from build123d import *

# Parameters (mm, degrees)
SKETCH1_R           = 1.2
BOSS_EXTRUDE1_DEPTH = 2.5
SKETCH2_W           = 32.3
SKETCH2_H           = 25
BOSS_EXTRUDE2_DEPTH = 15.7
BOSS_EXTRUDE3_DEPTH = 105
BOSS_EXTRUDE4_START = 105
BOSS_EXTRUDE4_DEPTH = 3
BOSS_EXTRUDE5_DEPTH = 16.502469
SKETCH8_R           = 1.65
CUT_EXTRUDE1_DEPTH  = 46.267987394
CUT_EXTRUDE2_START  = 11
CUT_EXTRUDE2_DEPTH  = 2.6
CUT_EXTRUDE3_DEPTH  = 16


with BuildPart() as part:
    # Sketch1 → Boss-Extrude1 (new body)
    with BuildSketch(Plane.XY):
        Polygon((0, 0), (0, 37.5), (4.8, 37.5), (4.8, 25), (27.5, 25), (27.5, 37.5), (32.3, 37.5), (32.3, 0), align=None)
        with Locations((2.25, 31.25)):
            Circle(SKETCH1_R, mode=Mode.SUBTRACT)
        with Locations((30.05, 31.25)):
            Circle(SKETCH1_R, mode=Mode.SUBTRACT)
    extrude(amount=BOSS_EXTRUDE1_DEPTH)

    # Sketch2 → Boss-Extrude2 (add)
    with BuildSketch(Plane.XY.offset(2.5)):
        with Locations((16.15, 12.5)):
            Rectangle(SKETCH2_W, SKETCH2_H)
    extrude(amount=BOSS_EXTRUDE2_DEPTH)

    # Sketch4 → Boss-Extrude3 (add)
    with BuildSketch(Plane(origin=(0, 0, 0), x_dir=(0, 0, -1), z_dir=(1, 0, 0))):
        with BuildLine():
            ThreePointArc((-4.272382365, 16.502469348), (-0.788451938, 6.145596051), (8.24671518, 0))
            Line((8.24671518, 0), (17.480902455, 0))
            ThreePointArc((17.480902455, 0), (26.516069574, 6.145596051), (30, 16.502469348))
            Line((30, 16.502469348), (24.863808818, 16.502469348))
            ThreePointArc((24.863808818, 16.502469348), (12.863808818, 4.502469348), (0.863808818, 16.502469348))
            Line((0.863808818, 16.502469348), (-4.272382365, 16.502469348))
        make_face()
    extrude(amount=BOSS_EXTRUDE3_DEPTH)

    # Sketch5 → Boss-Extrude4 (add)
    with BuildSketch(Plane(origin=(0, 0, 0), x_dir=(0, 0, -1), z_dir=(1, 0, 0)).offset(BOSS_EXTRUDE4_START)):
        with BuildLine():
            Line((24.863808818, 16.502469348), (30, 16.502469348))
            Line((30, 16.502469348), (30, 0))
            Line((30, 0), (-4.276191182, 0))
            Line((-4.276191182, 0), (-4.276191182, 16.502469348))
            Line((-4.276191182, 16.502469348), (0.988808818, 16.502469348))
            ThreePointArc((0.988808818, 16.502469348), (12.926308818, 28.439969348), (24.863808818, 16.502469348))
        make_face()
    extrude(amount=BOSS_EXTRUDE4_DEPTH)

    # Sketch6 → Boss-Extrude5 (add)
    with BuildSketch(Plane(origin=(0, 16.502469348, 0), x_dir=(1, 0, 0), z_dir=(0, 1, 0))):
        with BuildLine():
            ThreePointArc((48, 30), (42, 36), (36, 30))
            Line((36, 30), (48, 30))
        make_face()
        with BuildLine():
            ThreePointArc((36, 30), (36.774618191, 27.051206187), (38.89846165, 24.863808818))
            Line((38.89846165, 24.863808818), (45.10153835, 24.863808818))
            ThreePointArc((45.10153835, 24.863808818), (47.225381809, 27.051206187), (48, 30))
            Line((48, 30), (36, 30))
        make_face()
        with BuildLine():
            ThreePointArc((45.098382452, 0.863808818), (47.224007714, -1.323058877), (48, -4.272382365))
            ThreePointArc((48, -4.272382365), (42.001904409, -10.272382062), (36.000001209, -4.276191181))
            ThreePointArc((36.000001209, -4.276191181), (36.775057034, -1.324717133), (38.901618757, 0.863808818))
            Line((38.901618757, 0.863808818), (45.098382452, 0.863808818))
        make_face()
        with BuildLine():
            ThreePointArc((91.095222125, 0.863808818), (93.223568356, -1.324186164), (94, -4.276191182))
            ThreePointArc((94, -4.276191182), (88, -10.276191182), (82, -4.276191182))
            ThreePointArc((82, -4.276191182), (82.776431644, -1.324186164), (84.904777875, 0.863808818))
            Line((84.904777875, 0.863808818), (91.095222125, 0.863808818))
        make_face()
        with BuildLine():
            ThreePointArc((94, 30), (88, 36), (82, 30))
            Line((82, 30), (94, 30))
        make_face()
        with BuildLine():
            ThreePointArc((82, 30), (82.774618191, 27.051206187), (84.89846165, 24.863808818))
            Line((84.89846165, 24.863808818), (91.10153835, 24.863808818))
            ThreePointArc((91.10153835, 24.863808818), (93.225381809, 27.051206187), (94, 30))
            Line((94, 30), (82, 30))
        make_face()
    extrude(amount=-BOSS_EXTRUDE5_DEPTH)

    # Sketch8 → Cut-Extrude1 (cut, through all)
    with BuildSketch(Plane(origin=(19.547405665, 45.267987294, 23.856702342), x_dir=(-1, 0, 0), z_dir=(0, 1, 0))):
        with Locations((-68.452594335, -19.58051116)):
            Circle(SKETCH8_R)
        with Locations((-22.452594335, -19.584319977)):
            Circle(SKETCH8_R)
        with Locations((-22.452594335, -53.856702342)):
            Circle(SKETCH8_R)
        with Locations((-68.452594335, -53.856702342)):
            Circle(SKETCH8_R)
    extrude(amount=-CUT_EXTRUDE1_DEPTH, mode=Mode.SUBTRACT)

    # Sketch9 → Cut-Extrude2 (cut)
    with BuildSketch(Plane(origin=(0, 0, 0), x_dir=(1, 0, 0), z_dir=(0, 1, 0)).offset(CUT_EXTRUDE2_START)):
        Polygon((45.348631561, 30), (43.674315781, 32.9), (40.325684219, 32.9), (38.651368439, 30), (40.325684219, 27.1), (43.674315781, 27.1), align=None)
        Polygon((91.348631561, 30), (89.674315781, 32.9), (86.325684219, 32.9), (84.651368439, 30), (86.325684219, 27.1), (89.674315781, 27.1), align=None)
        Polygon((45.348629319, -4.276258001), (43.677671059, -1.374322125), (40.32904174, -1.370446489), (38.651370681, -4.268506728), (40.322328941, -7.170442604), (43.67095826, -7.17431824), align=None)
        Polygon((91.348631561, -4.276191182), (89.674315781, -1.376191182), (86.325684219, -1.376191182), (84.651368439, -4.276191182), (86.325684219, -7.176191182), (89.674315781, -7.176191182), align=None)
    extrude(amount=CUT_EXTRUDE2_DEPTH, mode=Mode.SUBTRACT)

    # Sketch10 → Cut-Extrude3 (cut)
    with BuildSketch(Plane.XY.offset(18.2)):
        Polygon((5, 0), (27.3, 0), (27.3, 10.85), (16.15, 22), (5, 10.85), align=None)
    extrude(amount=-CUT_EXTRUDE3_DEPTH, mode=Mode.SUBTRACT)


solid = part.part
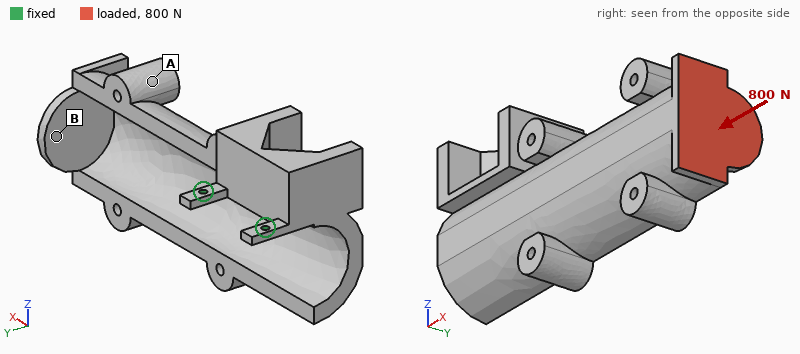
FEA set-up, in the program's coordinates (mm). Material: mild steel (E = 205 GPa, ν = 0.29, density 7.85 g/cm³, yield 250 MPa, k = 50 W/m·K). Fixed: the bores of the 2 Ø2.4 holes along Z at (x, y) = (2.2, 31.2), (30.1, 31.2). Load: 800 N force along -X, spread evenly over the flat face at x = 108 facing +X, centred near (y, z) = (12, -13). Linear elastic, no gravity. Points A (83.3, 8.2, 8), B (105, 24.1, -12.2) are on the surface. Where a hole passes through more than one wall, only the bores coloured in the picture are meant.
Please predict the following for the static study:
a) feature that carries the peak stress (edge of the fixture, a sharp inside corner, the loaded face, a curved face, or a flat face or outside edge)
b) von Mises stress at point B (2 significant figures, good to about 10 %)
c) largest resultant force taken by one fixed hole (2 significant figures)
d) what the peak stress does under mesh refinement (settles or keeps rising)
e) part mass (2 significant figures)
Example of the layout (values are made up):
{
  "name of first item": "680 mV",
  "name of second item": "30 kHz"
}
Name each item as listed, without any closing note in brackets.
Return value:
{
  "feature that carries the peak stress": "edge of the fixture",
  "von Mises stress at point B": "23 MPa",
  "largest resultant force taken by one fixed hole": "720 N",
  "what the peak stress does under mesh refinement": "keeps rising",
  "part mass": "310 g"
}
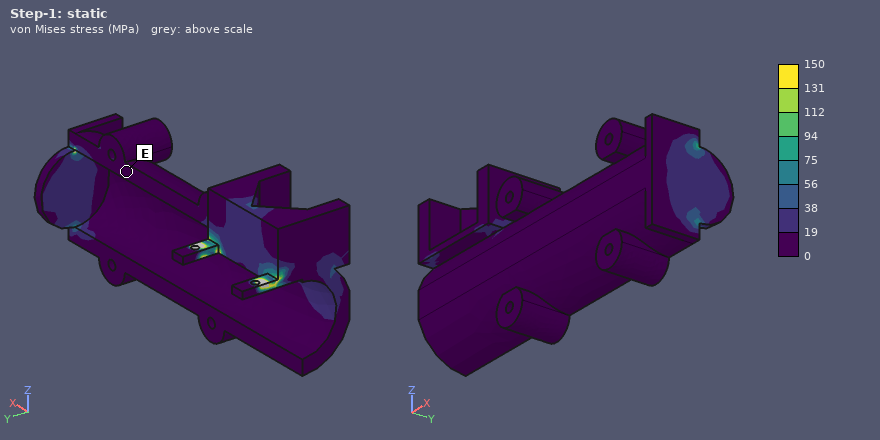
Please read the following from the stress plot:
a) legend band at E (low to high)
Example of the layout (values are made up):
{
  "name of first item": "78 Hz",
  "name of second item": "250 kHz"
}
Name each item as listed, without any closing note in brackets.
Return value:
{
  "legend band at E": "0 to 19 MPa"
}
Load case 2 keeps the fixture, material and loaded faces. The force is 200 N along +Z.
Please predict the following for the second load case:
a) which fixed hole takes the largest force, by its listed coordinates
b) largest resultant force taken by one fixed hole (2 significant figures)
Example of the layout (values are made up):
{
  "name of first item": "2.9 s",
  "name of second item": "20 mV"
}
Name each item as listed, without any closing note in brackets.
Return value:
{
  "which fixed hole takes the largest force, by its listed coordinates": "(30.1, 31.2)",
  "largest resultant force taken by one fixed hole": "750 N"
}
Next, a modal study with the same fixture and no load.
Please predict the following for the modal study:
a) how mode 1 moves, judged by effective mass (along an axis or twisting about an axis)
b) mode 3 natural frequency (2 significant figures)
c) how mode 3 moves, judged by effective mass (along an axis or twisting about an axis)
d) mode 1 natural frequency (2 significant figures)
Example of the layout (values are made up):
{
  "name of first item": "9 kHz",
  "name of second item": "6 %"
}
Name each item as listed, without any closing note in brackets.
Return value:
{
  "how mode 1 moves, judged by effective mass": "along Z",
  "mode 3 natural frequency": "940 Hz",
  "how mode 3 moves, judged by effective mass": "along Y",
  "mode 1 natural frequency": "210 Hz"
}
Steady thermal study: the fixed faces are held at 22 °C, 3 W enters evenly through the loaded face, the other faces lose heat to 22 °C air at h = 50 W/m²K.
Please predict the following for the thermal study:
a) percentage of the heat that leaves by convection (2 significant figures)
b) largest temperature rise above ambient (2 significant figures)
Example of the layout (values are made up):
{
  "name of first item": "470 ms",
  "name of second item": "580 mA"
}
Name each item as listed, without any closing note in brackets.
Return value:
{
  "percentage of the heat that leaves by convection": "96 %",
  "largest temperature rise above ambient": "12 K"
}
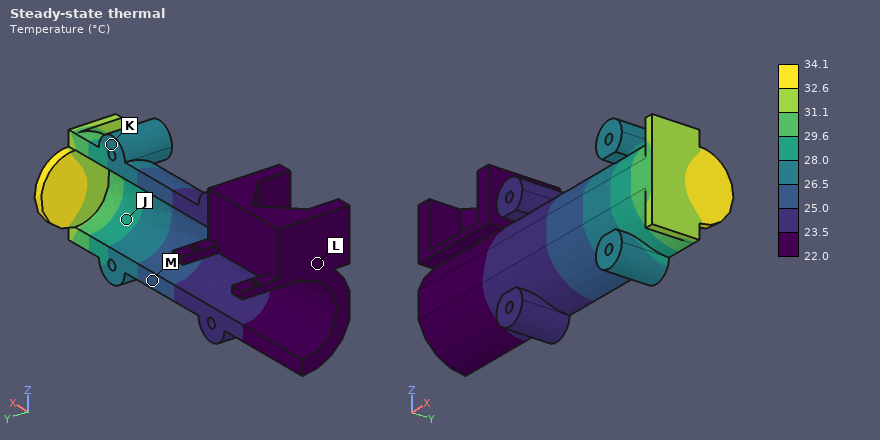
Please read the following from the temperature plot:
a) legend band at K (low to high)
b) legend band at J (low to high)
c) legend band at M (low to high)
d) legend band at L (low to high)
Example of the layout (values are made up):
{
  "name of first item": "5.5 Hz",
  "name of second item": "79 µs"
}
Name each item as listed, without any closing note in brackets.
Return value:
{
  "legend band at K": "26.5 to 28.0 °C",
  "legend band at J": "28.0 to 29.6 °C",
  "legend band at M": "25.0 to 26.5 °C",
  "legend band at L": "22.0 to 23.5 °C"
}
